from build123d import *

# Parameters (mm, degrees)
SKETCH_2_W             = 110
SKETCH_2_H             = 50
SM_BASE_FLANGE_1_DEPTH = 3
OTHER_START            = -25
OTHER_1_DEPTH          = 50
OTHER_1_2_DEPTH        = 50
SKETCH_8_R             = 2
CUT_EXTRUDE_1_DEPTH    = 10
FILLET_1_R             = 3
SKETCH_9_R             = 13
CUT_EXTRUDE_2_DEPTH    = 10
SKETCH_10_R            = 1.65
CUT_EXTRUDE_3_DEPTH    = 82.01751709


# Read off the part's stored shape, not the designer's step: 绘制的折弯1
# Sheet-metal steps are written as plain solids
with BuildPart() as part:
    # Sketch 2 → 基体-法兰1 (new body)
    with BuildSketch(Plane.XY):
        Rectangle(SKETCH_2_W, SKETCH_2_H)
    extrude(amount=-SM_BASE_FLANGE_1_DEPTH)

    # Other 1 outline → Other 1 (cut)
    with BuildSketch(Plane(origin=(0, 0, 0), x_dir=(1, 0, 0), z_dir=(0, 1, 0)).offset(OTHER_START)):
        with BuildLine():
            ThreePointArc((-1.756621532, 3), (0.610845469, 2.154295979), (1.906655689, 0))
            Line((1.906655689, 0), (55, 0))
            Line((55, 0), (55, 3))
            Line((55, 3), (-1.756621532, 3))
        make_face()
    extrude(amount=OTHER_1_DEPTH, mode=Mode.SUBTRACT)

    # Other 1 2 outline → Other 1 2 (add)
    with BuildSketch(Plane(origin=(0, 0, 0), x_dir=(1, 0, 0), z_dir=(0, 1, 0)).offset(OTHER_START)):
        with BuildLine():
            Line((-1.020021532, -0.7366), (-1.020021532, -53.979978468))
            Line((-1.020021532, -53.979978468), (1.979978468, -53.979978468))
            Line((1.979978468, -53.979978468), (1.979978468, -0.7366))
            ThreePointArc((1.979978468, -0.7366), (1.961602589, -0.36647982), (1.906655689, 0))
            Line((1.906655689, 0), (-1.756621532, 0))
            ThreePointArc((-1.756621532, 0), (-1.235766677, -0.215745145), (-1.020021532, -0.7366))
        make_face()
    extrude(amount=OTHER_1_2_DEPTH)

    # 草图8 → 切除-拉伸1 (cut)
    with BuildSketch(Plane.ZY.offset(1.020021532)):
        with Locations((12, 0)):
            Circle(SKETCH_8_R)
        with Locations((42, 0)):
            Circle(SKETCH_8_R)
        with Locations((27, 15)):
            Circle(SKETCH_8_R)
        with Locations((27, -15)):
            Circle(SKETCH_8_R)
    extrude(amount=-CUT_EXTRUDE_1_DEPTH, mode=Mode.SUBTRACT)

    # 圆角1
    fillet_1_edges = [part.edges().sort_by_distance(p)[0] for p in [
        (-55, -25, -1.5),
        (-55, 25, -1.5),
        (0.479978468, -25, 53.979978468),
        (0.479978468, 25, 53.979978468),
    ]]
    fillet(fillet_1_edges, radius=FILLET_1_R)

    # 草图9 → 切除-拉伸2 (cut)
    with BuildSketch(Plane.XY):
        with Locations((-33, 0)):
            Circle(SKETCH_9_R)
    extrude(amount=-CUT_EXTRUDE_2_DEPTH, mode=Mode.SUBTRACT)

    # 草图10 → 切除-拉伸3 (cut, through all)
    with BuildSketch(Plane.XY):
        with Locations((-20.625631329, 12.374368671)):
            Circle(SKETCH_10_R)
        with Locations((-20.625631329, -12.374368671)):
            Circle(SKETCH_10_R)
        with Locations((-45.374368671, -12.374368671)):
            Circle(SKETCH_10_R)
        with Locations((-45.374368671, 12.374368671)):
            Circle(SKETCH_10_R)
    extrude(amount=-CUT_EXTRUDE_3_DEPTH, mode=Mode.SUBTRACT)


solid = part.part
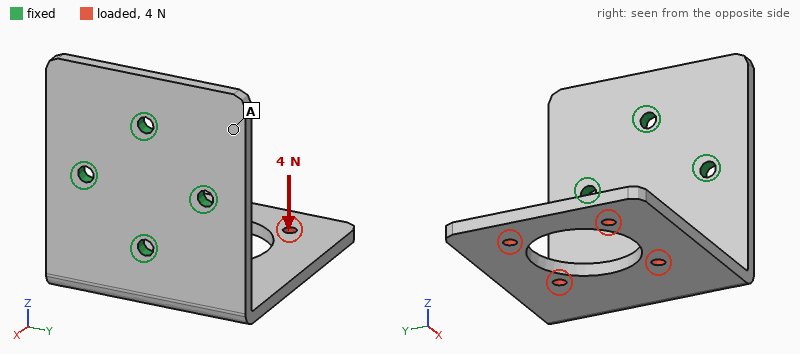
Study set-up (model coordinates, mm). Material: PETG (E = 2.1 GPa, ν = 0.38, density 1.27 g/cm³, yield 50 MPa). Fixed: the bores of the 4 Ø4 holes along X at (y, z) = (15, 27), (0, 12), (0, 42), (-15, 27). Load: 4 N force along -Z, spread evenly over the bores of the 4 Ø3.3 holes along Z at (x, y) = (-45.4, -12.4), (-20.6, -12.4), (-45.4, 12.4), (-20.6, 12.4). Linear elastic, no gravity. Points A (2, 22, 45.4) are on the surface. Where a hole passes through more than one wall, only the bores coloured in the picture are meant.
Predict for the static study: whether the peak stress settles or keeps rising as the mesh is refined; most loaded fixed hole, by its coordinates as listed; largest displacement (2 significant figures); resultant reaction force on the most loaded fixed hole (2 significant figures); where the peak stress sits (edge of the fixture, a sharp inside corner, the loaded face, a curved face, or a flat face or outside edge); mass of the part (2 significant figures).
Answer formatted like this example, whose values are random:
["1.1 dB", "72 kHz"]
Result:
["keeps rising", "(0, 12)", "0.92 mm", "5.7 N", "edge of the fixture", "19 g"]
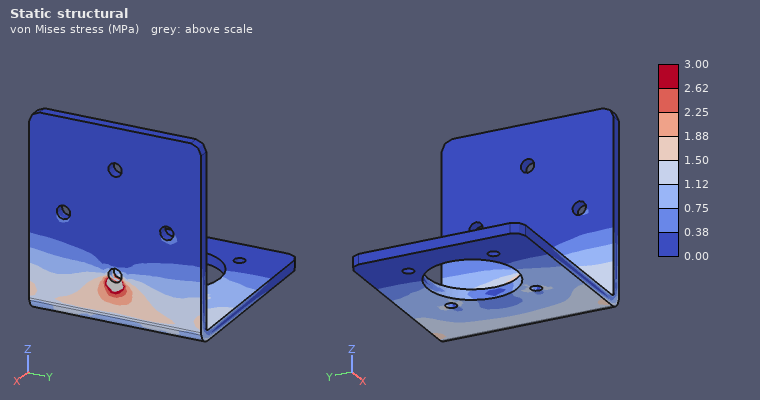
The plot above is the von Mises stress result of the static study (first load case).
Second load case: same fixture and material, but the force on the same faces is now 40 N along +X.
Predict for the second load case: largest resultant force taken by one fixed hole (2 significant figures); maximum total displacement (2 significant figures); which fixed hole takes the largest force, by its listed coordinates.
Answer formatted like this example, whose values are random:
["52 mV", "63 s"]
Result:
["51 N", "1.0 mm", "(0, 12)"]
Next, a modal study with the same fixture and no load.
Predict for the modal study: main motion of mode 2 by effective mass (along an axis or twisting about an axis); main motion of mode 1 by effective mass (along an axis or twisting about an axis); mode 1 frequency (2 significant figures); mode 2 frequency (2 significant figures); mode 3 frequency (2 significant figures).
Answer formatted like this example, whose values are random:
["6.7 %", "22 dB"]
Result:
["along Y", "along Z", "160 Hz", "270 Hz", "450 Hz"]
